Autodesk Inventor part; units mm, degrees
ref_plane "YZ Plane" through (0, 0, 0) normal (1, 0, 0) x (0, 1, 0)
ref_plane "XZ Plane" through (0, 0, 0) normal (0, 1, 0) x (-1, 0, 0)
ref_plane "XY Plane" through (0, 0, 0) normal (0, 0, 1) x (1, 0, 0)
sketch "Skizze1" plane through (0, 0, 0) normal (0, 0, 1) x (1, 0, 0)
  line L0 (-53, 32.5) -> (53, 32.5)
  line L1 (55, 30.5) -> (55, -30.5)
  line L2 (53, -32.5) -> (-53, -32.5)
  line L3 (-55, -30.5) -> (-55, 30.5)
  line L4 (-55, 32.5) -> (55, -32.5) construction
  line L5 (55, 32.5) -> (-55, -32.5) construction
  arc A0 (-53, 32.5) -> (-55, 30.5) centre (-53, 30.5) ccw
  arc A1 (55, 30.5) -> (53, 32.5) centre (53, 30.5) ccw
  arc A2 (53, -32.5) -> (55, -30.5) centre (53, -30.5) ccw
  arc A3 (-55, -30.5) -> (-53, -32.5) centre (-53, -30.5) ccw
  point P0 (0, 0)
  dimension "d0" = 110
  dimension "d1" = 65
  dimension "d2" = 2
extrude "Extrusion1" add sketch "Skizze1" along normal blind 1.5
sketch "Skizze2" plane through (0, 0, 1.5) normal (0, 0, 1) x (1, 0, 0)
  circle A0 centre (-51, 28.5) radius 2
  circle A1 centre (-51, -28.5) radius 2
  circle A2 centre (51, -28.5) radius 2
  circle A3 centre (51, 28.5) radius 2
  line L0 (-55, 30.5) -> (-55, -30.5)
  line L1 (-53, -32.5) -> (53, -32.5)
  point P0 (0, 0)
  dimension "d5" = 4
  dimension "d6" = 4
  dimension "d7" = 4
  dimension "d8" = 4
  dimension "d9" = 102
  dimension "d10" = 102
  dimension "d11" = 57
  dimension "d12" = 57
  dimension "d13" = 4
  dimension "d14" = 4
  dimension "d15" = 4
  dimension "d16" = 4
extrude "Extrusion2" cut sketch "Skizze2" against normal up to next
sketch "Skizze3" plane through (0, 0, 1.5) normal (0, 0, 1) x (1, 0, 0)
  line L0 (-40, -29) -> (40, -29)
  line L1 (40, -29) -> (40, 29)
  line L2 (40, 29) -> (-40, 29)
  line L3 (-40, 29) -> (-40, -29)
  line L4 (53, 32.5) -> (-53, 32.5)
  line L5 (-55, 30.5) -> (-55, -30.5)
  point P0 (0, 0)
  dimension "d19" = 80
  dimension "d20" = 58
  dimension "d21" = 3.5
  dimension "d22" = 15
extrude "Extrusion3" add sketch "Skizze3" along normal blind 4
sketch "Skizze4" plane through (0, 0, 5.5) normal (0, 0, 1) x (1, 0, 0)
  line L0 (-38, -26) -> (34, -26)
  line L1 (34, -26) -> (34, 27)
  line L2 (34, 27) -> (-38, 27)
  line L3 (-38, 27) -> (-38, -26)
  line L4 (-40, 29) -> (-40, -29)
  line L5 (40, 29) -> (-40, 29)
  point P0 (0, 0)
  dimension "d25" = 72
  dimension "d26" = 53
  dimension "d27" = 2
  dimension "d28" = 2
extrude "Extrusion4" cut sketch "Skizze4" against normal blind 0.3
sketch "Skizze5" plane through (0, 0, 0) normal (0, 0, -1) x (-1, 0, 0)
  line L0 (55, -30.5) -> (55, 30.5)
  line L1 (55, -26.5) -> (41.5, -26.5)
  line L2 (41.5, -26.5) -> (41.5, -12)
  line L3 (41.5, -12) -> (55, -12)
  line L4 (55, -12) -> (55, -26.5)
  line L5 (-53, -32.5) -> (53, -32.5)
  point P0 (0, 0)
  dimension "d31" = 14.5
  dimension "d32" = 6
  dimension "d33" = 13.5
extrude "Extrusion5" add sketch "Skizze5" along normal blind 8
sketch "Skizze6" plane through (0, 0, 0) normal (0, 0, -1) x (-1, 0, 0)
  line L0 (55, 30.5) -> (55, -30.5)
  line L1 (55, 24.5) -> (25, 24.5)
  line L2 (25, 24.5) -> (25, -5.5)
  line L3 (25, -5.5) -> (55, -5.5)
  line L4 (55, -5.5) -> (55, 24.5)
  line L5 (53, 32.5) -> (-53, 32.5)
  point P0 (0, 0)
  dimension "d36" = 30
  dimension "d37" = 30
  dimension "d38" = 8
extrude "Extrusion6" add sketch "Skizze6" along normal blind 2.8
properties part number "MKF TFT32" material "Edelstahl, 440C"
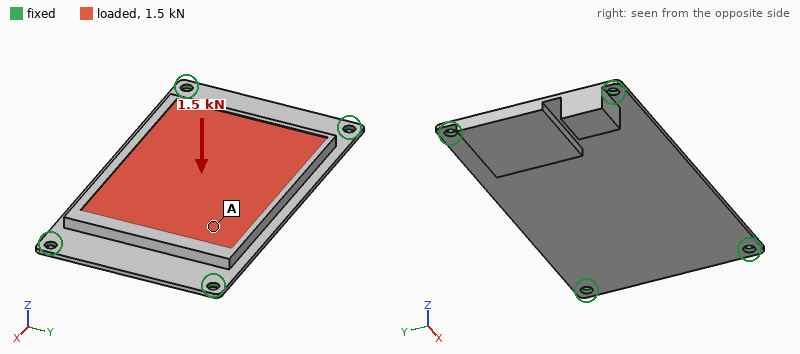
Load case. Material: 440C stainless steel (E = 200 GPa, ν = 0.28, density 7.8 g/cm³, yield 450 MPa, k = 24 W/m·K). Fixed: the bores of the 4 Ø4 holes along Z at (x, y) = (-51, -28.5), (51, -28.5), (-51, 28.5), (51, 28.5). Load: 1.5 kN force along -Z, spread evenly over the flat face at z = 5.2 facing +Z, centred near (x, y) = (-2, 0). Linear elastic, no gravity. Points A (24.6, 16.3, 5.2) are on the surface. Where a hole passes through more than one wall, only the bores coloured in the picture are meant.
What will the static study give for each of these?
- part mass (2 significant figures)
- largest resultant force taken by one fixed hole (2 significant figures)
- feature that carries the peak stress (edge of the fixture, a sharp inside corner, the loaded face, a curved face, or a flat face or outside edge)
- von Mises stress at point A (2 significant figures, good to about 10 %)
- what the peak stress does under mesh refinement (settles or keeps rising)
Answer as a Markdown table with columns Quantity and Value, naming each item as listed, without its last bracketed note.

| Quantity | Value |
|---|---|
| part mass | 250 g |
| largest resultant force taken by one fixed hole | 1.2 kN |
| feature that carries the peak stress | edge of the fixture |
| von Mises stress at point A | 42 MPa |
| what the peak stress does under mesh refinement | keeps rising |
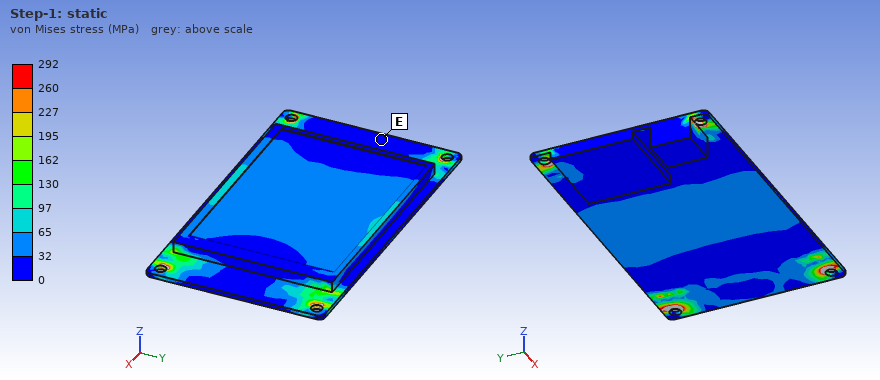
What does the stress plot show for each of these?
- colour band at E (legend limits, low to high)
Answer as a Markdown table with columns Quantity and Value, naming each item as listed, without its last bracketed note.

| Quantity | Value |
|---|---|
| colour band at E | 0 to 32 MPa |
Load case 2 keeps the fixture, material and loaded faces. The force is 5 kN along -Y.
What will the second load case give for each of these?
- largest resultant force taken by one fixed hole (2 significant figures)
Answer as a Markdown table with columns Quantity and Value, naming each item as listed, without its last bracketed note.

| Quantity | Value |
|---|---|
| largest resultant force taken by one fixed hole | 1.8 kN |
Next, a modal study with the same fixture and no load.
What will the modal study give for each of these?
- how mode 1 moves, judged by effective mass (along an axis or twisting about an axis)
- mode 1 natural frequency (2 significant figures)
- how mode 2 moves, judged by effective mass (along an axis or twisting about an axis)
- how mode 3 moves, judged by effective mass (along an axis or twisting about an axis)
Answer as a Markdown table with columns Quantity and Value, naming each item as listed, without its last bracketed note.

| Quantity | Value |
|---|---|
| how mode 1 moves, judged by effective mass | along Z |
| mode 1 natural frequency | 1400 Hz |
| how mode 2 moves, judged by effective mass | twisting about X |
| how mode 3 moves, judged by effective mass | twisting about Y |
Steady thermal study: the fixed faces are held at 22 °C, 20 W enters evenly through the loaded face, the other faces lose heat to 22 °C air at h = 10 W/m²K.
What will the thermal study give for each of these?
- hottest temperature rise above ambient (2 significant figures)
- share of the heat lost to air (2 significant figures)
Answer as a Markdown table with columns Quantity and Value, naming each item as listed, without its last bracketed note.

| Quantity | Value |
|---|---|
| hottest temperature rise above ambient | 78 K |
| share of the heat lost to air | 36 % |
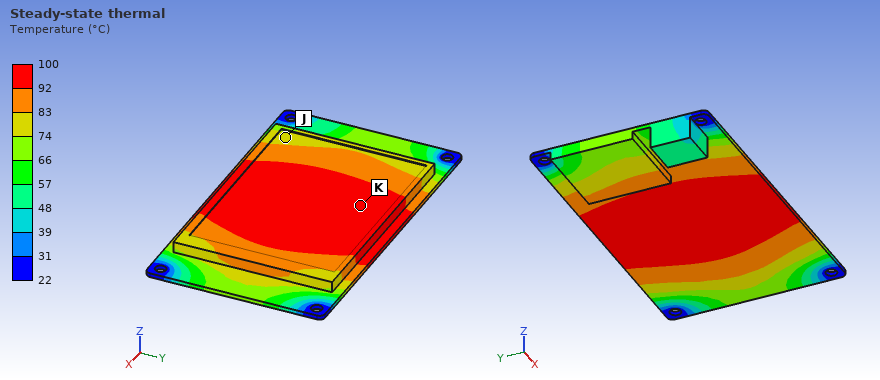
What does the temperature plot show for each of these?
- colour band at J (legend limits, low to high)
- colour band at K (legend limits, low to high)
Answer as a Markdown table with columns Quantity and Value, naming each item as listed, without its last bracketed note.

| Quantity | Value |
|---|---|
| colour band at J | 74 to 83 °C |
| colour band at K | 92 to 100 °C |
